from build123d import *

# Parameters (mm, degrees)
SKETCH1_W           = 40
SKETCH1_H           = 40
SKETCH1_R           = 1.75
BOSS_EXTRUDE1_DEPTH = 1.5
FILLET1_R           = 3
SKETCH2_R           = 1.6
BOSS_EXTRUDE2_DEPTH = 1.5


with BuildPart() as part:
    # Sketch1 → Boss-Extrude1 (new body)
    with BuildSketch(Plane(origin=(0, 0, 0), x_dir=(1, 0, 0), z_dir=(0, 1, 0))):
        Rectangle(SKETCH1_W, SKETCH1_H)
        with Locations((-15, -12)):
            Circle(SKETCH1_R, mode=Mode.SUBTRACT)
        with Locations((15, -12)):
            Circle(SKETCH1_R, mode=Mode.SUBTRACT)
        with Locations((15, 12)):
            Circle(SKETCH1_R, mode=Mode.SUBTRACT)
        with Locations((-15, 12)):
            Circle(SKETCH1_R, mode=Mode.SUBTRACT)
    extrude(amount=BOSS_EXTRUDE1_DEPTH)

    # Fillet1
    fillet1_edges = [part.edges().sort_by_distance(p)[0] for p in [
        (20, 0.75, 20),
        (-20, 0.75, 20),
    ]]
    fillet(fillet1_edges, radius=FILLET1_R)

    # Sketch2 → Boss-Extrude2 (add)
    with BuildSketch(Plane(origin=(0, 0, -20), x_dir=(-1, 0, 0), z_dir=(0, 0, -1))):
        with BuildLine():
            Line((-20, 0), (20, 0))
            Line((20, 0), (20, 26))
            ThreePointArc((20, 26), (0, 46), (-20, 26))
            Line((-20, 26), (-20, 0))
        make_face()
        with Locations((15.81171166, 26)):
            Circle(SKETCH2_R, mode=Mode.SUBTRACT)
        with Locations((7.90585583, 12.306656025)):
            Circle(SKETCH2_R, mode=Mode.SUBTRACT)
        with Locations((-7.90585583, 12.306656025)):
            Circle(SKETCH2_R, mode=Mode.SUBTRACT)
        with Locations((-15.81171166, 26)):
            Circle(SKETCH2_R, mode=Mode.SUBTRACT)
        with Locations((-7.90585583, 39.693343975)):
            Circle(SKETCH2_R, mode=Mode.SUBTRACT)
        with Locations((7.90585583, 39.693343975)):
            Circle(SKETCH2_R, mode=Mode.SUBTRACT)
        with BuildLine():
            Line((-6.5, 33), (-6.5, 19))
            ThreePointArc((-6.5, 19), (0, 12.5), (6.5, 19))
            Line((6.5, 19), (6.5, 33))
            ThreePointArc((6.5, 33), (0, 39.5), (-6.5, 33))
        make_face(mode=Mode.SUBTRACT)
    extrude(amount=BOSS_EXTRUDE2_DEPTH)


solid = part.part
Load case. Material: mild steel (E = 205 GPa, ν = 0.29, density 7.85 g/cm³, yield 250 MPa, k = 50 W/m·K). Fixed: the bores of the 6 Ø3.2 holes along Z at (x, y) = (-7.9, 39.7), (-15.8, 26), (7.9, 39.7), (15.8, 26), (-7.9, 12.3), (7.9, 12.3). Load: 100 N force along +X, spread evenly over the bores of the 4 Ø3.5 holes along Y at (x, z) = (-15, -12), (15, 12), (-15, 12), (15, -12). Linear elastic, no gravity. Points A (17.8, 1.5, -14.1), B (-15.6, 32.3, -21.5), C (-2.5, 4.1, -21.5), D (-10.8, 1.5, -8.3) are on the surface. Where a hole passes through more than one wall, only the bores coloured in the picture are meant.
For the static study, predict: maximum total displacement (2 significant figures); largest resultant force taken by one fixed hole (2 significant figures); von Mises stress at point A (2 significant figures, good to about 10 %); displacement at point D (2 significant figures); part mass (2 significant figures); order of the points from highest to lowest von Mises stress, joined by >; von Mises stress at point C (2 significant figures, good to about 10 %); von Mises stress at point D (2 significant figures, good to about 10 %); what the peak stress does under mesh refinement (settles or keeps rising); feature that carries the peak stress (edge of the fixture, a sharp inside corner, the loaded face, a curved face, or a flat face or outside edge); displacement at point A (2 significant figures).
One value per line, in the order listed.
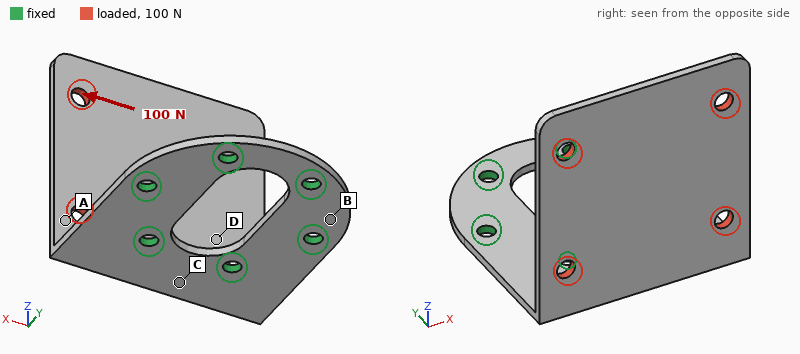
0.10 mm
120 N
30 MPa
0.039 mm
34 g
C > A > D > B
48 MPa
14 MPa
keeps rising
edge of the fixture
0.042 mm
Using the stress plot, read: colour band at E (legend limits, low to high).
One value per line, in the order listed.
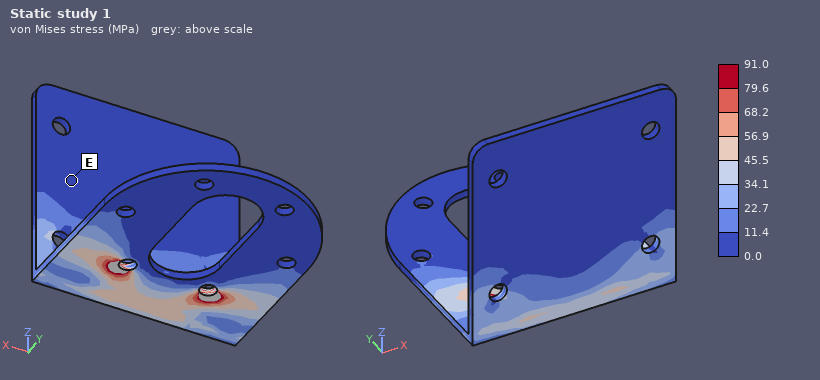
0.0 to 11.4 MPa
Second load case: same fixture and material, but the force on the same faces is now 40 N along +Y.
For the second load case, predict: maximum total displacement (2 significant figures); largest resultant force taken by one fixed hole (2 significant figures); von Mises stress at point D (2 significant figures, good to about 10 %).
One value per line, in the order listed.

0.30 mm
19 N
25 MPa
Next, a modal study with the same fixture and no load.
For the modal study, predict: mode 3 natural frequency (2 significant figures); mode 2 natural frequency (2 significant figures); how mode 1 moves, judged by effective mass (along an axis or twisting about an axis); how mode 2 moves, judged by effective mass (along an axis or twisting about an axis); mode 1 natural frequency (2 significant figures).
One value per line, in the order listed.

1900 Hz
1300 Hz
along Y
along X
530 Hz
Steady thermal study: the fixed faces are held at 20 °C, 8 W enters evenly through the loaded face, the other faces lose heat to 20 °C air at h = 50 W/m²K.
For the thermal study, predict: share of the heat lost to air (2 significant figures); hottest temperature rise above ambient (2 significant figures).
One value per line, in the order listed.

63 %
42 K
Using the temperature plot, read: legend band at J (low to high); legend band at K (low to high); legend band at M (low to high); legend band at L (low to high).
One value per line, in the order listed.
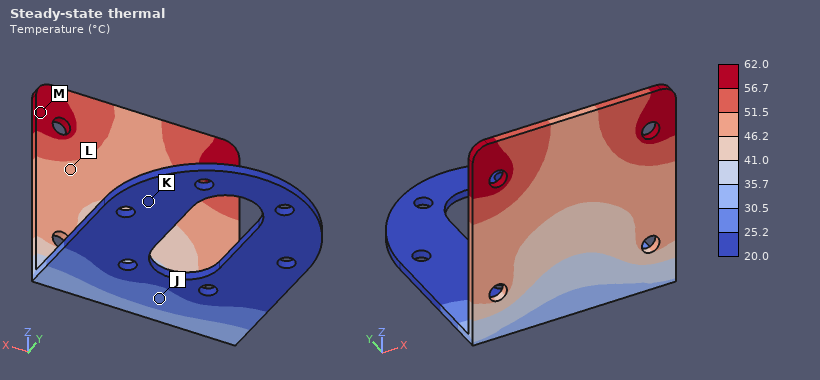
25.2 to 30.5 °C
20.0 to 25.2 °C
56.7 to 62.0 °C
46.2 to 51.5 °C
